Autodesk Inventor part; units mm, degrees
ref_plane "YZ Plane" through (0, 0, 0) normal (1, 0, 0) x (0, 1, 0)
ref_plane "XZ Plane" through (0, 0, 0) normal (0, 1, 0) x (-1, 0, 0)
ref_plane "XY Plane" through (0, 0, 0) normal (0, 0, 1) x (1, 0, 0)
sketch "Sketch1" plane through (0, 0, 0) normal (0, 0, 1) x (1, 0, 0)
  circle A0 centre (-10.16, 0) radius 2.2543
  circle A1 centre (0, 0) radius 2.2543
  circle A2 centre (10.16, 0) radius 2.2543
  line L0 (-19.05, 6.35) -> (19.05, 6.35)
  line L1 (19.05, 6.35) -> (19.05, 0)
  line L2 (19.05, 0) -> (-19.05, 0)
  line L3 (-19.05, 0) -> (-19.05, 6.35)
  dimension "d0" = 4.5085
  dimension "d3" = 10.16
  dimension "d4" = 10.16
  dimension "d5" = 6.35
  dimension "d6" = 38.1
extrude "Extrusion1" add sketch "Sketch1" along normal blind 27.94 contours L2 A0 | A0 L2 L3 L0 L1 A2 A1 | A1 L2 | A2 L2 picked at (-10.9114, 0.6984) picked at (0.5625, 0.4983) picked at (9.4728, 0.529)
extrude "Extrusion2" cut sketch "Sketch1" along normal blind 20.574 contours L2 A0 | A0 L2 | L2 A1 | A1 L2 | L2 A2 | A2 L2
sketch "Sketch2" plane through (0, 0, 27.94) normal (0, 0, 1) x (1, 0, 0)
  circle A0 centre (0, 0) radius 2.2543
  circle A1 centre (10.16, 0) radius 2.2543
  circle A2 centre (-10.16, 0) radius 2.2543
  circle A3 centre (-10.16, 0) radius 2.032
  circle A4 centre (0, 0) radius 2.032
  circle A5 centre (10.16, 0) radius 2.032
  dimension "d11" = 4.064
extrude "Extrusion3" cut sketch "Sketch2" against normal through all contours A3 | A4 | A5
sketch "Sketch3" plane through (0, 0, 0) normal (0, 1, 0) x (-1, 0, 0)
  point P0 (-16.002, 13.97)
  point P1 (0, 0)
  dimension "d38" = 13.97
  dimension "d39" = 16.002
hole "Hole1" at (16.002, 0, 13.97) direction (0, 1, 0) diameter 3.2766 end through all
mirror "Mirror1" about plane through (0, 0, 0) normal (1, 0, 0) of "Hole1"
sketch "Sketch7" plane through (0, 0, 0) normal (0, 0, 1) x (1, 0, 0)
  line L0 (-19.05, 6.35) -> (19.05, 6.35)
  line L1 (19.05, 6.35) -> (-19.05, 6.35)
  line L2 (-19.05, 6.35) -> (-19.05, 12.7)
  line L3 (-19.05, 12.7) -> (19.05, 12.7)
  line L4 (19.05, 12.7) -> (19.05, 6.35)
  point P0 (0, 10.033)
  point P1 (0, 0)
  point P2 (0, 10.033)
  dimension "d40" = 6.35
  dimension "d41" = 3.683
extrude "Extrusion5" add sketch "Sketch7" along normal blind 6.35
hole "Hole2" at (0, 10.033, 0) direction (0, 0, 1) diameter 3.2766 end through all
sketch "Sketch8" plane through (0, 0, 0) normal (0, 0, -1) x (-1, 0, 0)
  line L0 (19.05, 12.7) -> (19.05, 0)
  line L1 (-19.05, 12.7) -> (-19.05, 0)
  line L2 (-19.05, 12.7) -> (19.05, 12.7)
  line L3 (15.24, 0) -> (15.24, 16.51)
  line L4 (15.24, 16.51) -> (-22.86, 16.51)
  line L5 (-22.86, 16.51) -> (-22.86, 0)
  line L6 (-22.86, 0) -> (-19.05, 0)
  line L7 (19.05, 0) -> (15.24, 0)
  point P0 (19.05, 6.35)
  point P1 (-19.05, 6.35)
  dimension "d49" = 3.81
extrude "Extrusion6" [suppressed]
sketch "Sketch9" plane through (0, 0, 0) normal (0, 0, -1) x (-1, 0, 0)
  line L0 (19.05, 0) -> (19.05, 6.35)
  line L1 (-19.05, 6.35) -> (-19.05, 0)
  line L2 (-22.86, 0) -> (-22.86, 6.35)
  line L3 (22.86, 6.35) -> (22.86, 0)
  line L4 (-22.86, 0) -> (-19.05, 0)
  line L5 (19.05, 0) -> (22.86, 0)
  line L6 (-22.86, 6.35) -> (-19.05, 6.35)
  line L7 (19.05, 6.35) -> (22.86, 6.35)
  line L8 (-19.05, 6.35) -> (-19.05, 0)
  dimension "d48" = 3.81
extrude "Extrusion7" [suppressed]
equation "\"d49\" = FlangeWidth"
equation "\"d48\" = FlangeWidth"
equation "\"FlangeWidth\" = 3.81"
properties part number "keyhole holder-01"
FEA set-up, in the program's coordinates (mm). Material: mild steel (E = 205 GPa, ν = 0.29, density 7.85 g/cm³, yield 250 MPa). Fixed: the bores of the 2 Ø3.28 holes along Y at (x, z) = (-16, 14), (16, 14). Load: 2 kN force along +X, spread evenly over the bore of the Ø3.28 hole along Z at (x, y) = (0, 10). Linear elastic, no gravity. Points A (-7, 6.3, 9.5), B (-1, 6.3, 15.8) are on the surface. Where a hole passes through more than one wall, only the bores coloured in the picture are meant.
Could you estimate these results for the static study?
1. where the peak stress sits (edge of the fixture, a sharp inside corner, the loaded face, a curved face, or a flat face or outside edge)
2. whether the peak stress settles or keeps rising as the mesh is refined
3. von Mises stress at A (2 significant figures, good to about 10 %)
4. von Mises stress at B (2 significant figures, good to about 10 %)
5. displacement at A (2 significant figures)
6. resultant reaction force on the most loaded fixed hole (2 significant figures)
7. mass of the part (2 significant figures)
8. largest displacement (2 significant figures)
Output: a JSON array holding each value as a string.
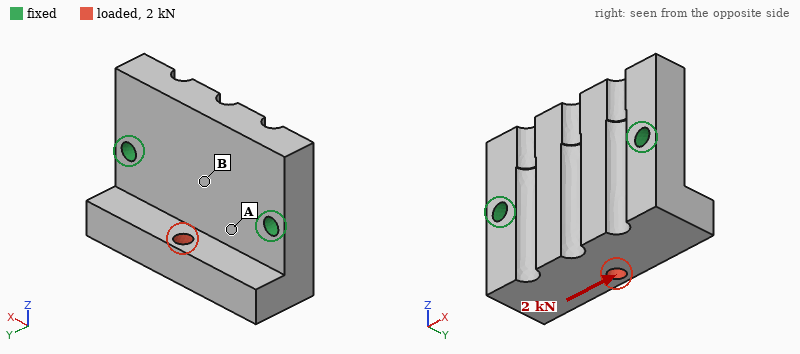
["edge of the fixture", "keeps rising", "31 MPa", "10 MPa", "1.3 µm", "1.2 kN", "59 g", "5.0 µm"]
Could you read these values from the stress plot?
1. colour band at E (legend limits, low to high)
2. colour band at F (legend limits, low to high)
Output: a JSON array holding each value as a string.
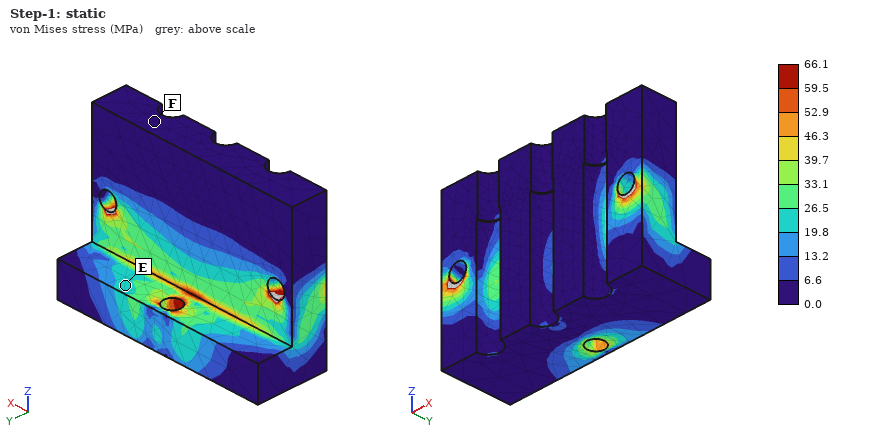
["19.8 to 26.5 MPa", "0.0 to 6.6 MPa"]
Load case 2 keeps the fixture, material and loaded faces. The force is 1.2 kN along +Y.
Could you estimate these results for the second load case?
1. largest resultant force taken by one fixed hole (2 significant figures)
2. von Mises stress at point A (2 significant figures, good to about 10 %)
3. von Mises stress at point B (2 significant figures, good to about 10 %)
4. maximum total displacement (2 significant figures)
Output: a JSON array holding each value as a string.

["620 N", "22 MPa", "21 MPa", "15 µm"]
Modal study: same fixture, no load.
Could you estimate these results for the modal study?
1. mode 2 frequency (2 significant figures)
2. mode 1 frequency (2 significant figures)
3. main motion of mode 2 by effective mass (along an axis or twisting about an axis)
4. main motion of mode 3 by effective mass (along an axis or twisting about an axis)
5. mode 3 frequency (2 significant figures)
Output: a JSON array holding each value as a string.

["16 kHz", "11 kHz", "along Y", "twisting about Z", "20 kHz"]
